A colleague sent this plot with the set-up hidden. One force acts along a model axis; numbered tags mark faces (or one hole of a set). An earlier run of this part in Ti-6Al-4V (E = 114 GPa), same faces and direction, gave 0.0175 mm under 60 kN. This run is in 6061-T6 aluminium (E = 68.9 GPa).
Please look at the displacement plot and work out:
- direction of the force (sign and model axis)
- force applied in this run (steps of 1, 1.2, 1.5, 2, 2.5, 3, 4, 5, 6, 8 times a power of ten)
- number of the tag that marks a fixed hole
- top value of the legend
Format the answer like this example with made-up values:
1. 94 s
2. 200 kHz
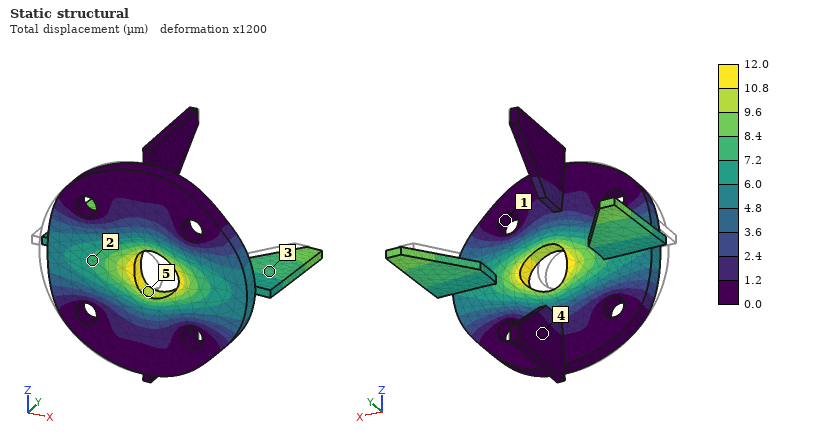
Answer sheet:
1. +X
2. 25 kN
3. 1
4. 12.0 µm
